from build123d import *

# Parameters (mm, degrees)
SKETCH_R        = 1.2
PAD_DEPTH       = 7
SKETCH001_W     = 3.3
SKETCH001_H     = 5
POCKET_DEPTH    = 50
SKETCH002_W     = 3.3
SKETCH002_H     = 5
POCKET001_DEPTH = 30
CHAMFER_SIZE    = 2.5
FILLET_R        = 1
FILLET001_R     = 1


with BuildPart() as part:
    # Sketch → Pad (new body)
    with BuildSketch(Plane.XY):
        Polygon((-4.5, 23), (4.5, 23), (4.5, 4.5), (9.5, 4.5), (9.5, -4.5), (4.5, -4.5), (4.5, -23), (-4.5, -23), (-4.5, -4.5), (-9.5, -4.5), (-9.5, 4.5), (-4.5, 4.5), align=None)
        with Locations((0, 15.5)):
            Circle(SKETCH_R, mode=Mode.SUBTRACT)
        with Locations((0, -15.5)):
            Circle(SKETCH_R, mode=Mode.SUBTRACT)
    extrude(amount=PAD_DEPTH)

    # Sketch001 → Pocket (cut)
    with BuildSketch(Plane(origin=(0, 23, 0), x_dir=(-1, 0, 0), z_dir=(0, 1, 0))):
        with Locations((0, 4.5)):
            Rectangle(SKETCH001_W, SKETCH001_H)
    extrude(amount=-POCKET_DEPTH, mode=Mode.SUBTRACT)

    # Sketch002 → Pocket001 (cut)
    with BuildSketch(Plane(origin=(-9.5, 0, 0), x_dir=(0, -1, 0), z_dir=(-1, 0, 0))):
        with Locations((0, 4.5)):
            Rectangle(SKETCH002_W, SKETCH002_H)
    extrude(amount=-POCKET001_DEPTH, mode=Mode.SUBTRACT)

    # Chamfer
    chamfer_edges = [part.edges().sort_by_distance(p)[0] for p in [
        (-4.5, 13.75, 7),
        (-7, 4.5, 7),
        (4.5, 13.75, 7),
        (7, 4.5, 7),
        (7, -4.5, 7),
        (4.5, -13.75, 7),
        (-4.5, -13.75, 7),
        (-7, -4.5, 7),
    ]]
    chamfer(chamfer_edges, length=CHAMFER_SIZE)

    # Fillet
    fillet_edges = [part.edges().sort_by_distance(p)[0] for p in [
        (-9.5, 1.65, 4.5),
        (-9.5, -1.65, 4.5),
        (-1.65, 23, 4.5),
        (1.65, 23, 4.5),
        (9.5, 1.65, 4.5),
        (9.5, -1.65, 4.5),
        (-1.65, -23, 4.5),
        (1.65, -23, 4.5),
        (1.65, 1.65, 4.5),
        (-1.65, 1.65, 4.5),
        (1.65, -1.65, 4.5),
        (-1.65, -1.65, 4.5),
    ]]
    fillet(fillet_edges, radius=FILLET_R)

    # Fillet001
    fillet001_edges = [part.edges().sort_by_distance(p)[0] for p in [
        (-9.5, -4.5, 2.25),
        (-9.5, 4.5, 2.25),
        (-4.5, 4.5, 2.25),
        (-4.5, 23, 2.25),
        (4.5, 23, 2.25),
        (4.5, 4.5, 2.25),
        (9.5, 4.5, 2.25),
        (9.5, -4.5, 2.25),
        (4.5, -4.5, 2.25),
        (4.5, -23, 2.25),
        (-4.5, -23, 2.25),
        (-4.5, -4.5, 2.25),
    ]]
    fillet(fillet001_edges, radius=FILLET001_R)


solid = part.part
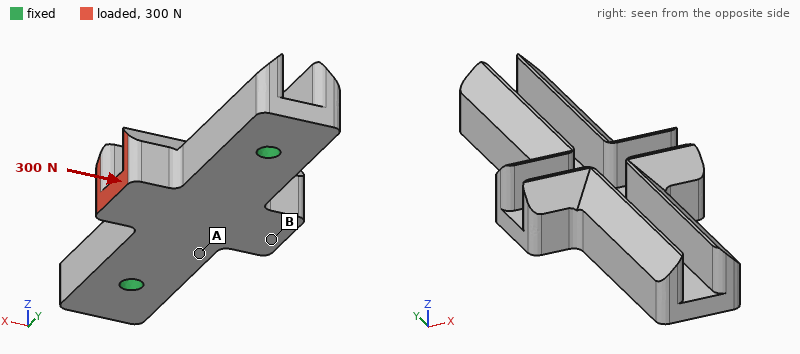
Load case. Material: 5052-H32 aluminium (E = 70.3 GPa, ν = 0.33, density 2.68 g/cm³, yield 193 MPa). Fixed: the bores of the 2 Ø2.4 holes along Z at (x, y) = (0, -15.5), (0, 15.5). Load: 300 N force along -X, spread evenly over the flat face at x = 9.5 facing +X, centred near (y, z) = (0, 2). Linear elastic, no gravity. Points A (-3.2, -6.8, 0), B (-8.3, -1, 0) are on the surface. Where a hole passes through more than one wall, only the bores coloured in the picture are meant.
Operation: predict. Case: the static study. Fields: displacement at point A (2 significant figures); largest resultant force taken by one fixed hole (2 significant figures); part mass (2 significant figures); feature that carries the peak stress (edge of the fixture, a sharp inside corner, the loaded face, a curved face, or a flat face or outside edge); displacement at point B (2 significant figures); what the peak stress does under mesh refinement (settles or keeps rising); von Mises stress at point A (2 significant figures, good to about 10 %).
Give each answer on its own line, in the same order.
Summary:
6.0 µm
150 N
5.8 g
edge of the fixture
7.2 µm
keeps rising
16 MPa
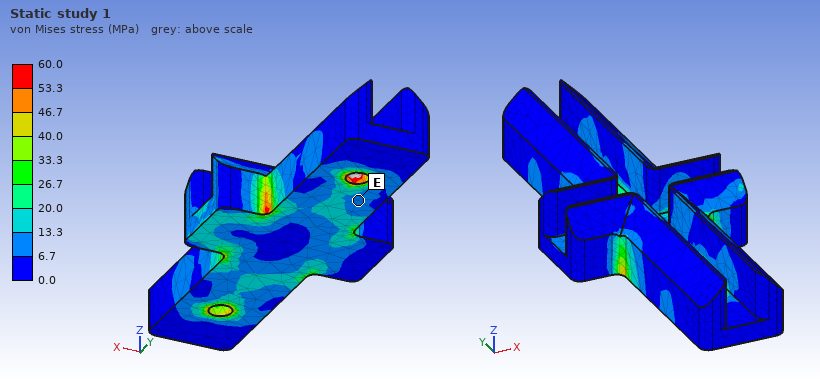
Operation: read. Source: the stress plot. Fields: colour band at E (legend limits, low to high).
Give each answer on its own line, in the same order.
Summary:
6.7 to 13.3 MPa
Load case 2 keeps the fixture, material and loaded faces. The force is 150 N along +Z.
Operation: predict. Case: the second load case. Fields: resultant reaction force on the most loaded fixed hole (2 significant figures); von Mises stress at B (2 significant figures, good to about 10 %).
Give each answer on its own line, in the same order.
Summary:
77 N
11 MPa
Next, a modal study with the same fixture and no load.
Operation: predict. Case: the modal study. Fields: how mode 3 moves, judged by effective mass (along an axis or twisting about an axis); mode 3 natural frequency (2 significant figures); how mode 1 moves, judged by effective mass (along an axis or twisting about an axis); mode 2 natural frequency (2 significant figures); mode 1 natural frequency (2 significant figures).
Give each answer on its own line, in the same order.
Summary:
along X
19 kHz
along Z
10 kHz
9100 Hz
